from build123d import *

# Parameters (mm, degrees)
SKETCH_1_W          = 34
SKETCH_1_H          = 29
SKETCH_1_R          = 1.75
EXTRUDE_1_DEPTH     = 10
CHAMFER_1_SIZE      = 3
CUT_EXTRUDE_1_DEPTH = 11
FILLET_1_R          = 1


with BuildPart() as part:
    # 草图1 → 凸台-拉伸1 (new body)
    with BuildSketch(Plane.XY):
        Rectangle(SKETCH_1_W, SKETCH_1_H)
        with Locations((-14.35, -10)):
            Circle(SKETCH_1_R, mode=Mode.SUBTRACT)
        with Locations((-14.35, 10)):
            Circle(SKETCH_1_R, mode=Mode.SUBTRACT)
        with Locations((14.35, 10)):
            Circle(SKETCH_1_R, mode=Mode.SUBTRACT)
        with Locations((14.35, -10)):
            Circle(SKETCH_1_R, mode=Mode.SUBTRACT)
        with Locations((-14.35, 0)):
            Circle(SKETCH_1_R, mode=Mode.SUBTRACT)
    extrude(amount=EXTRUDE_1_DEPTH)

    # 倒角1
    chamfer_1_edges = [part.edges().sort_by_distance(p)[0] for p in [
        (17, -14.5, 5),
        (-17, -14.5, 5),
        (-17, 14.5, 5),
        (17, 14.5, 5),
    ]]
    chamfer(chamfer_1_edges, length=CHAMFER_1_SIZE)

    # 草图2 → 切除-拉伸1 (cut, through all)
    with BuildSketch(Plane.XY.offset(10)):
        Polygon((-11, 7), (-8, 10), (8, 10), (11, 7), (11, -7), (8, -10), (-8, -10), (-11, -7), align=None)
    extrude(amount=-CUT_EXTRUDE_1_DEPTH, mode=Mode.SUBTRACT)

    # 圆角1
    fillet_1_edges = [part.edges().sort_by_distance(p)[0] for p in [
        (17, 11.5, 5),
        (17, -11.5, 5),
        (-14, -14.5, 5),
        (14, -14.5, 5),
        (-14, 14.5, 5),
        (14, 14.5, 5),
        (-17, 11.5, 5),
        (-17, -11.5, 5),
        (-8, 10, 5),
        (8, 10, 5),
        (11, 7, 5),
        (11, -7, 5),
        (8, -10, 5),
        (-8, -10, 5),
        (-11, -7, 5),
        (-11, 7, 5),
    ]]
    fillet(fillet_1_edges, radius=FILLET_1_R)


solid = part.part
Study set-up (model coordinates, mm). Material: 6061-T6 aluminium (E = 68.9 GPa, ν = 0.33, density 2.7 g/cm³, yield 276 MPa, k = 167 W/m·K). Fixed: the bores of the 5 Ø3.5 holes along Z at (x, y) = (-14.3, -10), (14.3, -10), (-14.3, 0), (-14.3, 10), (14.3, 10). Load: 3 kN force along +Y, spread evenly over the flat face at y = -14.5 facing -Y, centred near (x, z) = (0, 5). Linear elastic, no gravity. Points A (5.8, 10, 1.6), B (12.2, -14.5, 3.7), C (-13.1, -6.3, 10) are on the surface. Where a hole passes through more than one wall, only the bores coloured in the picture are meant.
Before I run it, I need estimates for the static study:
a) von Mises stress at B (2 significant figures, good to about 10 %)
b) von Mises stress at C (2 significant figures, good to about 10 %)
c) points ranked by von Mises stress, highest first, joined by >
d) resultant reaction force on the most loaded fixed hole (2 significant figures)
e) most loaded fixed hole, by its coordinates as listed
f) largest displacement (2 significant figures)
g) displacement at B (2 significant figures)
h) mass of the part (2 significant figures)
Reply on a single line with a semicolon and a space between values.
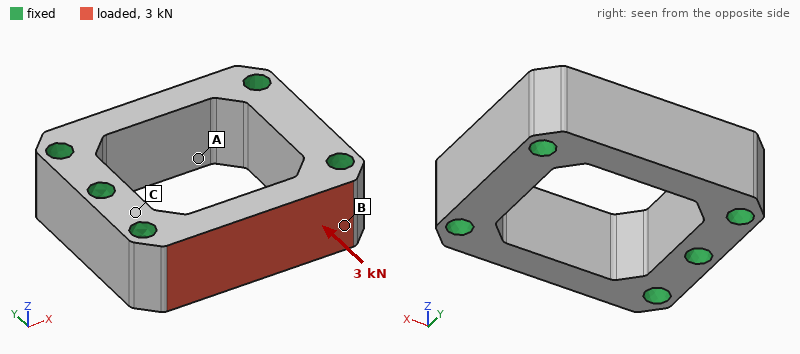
37 MPa; 23 MPa; B > C > A; 1.5 kN; (14.3, -10); 23 µm; 4.4 µm; 13 g
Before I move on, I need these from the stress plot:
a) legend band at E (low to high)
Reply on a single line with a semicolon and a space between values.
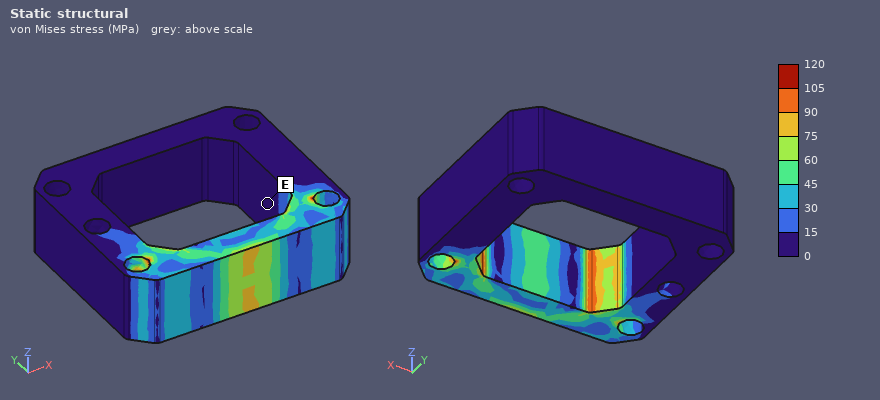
0 to 15 MPa
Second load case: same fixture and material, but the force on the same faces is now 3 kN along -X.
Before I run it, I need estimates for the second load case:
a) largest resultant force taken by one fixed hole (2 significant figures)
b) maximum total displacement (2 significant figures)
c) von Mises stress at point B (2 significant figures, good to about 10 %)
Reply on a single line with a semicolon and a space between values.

1.6 kN; 3.9 µm; 24 MPa
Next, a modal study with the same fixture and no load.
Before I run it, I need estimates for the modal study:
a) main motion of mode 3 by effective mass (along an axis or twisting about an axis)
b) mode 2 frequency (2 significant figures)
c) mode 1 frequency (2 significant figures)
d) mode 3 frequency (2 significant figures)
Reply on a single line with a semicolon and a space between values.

along Z; 37 kHz; 36 kHz; 46 kHz
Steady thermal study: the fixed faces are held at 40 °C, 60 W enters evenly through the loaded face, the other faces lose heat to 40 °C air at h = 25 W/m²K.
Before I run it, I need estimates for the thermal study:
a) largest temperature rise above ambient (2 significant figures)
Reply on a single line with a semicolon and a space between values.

25 K
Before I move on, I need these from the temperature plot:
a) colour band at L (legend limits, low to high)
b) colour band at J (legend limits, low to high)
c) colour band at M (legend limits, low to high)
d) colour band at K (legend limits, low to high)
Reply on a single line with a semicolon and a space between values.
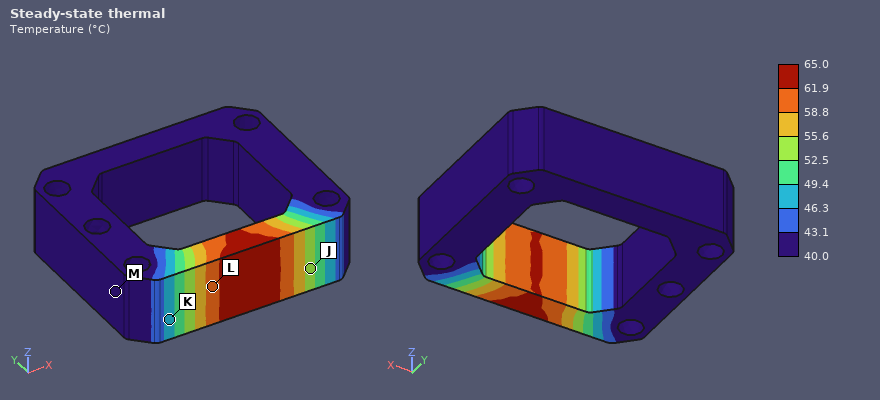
58.8 to 61.9 °C; 52.5 to 55.6 °C; 40.0 to 43.1 °C; 46.3 to 49.4 °C
